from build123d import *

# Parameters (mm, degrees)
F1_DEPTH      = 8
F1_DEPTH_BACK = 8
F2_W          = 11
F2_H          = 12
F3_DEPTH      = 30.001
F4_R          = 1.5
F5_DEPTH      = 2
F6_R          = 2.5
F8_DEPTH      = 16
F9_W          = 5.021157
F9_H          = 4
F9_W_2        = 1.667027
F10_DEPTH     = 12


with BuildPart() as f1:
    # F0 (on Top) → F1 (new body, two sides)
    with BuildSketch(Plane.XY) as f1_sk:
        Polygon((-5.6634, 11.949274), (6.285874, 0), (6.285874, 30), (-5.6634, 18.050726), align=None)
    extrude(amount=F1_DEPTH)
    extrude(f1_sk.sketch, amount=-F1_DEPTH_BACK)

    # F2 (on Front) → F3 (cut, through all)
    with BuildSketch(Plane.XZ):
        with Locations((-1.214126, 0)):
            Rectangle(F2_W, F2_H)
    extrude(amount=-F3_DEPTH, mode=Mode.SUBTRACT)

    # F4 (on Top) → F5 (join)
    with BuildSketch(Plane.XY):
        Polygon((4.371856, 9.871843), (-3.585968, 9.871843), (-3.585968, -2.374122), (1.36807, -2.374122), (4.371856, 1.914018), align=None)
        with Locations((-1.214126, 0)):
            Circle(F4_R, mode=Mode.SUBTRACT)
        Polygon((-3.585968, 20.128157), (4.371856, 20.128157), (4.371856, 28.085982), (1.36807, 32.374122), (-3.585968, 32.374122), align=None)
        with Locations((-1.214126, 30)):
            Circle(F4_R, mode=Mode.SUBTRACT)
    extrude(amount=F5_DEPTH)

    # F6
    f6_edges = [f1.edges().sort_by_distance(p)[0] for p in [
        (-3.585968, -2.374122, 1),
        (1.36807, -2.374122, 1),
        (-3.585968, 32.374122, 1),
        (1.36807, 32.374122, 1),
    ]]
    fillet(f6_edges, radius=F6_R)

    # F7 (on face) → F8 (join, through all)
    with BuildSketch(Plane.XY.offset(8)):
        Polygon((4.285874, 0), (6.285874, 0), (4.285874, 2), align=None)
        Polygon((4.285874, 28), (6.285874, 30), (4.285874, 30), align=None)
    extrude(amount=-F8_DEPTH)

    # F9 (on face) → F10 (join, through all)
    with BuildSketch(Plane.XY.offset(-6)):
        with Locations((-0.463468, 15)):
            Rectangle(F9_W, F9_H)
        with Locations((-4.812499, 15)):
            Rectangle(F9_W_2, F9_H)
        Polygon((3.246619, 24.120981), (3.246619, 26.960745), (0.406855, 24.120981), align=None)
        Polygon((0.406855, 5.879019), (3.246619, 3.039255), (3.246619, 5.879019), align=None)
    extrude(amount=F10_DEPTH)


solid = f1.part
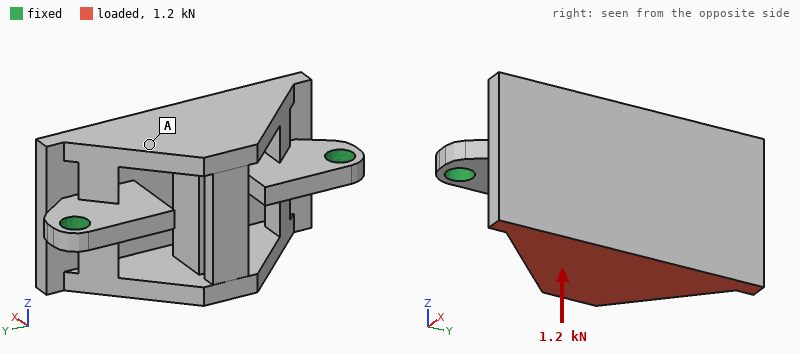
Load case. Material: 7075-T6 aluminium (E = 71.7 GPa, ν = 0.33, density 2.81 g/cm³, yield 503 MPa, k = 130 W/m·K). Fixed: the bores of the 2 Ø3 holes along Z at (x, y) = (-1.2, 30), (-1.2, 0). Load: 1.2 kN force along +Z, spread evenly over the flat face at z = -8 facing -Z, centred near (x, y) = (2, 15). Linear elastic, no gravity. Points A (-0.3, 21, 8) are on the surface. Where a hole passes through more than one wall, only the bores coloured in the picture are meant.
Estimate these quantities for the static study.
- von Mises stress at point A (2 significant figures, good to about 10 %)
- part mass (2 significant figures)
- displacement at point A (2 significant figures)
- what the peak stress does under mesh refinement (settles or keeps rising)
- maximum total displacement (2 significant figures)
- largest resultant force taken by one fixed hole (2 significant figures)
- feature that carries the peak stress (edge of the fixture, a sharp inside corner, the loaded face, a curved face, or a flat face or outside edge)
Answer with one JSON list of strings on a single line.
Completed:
["30 MPa", "6.5 g", "45 µm", "keeps rising", "57 µm", "600 N", "edge of the fixture"]
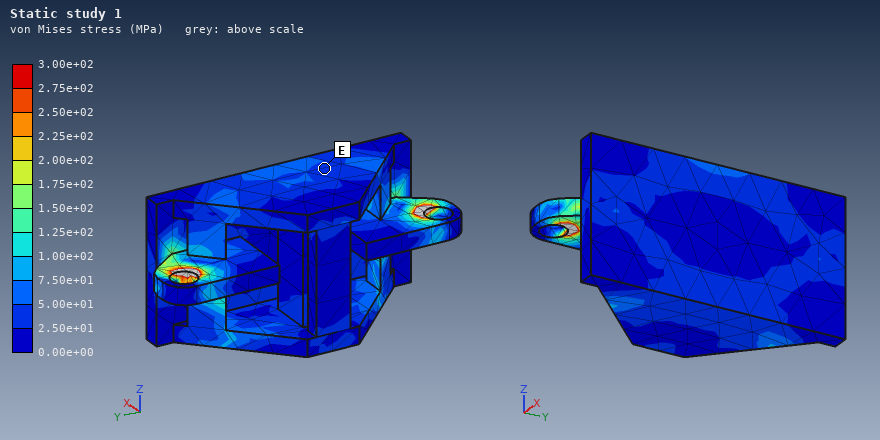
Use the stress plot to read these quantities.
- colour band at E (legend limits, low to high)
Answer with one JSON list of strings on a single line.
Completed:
["2.50e+01 to 5.00e+01 MPa"]
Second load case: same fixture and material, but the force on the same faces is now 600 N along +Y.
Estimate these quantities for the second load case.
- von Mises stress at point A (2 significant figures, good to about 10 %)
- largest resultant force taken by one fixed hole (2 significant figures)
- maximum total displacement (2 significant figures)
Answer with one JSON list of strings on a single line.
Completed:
["17 MPa", "360 N", "46 µm"]
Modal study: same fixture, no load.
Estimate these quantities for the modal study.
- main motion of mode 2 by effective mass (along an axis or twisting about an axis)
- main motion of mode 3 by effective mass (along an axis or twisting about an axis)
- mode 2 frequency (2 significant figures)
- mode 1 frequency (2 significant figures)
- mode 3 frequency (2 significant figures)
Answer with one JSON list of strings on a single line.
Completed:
["along Z", "along Y", "11 kHz", "4400 Hz", "13 kHz"]
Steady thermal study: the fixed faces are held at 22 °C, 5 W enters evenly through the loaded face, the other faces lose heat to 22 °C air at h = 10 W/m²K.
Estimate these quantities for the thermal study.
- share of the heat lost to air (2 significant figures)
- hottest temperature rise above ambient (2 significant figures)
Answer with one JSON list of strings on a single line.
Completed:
["4.2 %", "13 K"]
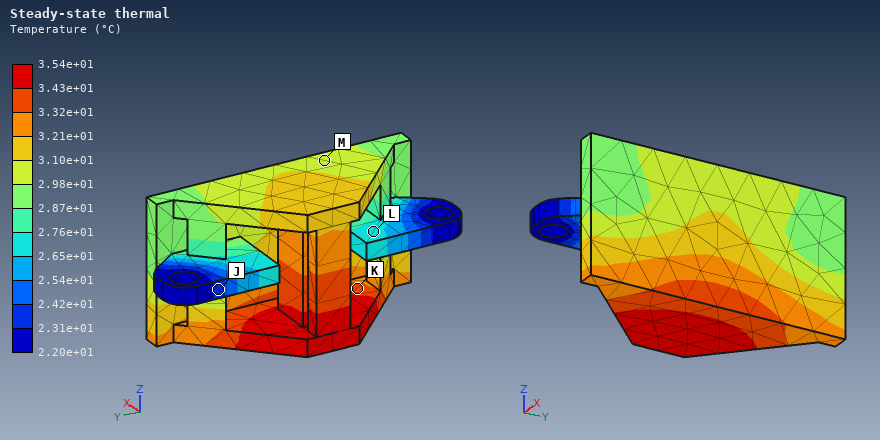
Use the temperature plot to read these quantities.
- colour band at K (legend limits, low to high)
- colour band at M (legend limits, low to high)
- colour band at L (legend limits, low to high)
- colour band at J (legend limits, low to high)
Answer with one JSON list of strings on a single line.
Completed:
["3.32e+01 to 3.43e+01 °C", "2.98e+01 to 3.10e+01 °C", "2.65e+01 to 2.76e+01 °C", "2.31e+01 to 2.42e+01 °C"]
